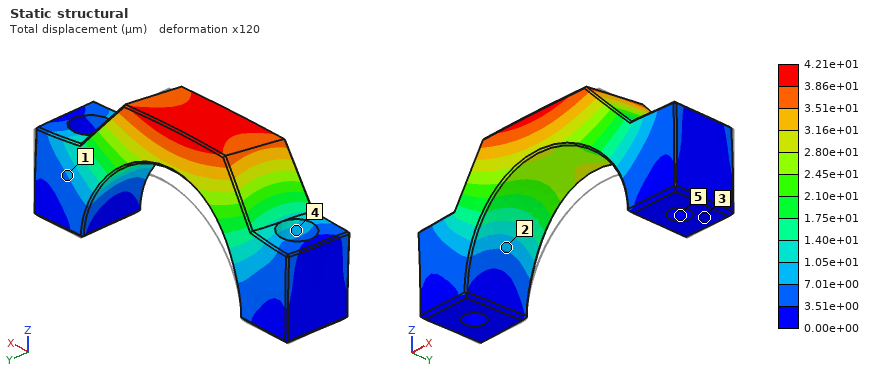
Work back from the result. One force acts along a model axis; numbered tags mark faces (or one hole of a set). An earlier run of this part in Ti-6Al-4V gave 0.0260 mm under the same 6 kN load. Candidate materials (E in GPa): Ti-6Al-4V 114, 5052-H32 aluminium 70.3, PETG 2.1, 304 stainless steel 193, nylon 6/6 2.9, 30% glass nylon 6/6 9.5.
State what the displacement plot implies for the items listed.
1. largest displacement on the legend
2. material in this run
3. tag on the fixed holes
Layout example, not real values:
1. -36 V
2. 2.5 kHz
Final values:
1. 4.21e+01 µm
2. 5052-H32 aluminium
3. 5
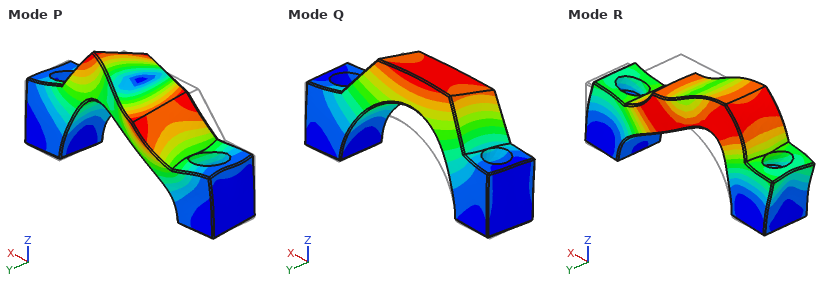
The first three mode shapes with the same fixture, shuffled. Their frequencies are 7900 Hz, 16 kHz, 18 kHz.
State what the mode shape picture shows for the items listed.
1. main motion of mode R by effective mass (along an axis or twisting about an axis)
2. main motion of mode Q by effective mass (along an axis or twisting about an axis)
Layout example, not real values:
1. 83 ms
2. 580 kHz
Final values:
1. along X
2. along Y
